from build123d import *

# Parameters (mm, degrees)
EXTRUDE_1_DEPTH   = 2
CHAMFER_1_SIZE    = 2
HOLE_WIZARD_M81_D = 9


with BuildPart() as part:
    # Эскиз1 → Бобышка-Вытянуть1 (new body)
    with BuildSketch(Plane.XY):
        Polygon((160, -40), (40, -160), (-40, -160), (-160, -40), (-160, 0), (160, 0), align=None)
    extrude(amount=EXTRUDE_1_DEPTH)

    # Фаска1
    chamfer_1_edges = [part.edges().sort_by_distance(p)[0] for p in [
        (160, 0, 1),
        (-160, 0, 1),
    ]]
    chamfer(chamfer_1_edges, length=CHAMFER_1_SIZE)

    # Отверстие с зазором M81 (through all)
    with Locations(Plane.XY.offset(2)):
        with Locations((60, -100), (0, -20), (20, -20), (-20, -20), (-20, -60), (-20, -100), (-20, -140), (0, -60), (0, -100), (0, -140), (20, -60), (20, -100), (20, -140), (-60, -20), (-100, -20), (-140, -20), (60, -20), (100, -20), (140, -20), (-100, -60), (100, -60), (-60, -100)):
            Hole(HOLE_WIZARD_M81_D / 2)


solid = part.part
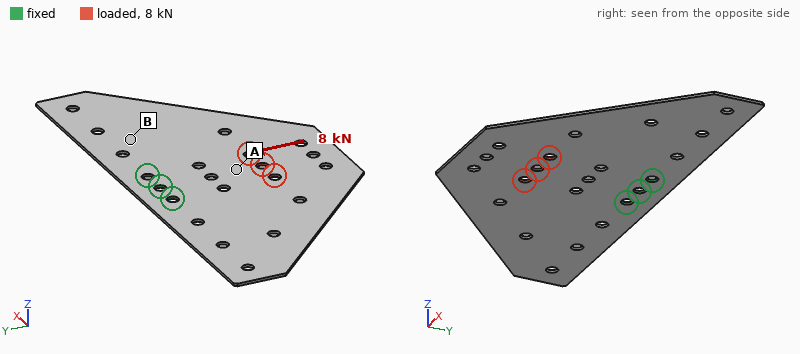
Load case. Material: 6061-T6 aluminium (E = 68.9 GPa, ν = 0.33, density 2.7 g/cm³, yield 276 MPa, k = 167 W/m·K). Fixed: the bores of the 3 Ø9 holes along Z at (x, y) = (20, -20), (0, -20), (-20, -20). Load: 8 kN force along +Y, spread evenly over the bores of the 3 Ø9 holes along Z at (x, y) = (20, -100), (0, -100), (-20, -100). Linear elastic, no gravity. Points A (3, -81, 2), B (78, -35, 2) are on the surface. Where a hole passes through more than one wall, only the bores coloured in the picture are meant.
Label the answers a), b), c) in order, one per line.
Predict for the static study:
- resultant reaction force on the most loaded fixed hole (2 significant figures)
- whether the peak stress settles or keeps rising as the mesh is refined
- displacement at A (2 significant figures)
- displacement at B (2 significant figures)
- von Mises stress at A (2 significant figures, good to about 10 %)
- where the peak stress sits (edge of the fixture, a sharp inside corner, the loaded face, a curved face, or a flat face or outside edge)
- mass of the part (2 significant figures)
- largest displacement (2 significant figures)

a) 3.2 kN
b) keeps rising
c) 50 µm
d) 37 µm
e) 54 MPa
f) a sharp inside corner
g) 190 g
h) 70 µm
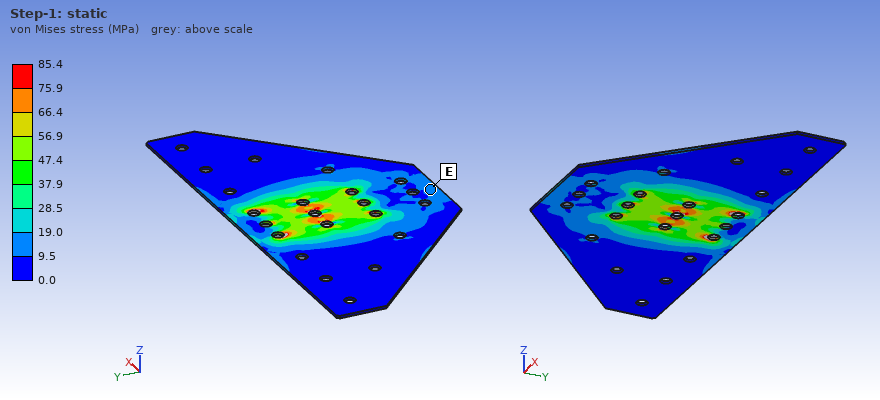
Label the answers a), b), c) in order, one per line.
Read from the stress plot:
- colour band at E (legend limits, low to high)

a) 9.5 to 19.0 MPa
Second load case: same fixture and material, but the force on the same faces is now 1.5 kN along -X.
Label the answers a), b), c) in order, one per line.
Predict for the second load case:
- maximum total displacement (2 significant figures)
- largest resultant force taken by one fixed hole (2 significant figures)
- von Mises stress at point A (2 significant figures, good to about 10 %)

a) 0.16 mm
b) 2.5 kN
c) 18 MPa
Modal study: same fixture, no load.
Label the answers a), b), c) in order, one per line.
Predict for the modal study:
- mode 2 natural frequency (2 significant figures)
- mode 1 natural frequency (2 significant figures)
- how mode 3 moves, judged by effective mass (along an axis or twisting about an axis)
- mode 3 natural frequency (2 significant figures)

a) 90 Hz
b) 89 Hz
c) along Z
d) 110 Hz
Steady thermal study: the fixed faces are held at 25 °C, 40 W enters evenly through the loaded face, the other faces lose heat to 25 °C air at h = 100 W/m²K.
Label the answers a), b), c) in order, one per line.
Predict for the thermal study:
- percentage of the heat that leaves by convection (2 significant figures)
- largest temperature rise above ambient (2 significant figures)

a) 90 %
b) 31 K
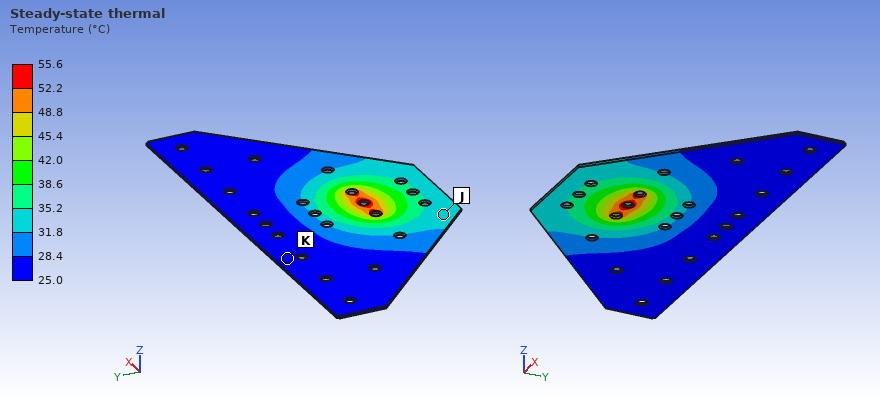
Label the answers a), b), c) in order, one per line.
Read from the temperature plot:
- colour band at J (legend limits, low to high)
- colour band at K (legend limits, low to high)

a) 31.8 to 35.2 °C
b) 25.0 to 28.4 °C
